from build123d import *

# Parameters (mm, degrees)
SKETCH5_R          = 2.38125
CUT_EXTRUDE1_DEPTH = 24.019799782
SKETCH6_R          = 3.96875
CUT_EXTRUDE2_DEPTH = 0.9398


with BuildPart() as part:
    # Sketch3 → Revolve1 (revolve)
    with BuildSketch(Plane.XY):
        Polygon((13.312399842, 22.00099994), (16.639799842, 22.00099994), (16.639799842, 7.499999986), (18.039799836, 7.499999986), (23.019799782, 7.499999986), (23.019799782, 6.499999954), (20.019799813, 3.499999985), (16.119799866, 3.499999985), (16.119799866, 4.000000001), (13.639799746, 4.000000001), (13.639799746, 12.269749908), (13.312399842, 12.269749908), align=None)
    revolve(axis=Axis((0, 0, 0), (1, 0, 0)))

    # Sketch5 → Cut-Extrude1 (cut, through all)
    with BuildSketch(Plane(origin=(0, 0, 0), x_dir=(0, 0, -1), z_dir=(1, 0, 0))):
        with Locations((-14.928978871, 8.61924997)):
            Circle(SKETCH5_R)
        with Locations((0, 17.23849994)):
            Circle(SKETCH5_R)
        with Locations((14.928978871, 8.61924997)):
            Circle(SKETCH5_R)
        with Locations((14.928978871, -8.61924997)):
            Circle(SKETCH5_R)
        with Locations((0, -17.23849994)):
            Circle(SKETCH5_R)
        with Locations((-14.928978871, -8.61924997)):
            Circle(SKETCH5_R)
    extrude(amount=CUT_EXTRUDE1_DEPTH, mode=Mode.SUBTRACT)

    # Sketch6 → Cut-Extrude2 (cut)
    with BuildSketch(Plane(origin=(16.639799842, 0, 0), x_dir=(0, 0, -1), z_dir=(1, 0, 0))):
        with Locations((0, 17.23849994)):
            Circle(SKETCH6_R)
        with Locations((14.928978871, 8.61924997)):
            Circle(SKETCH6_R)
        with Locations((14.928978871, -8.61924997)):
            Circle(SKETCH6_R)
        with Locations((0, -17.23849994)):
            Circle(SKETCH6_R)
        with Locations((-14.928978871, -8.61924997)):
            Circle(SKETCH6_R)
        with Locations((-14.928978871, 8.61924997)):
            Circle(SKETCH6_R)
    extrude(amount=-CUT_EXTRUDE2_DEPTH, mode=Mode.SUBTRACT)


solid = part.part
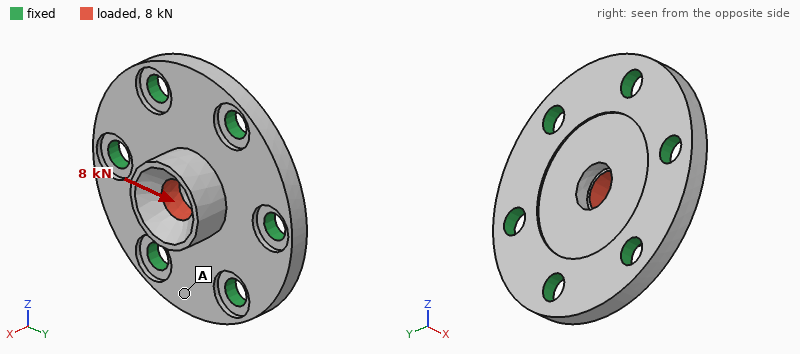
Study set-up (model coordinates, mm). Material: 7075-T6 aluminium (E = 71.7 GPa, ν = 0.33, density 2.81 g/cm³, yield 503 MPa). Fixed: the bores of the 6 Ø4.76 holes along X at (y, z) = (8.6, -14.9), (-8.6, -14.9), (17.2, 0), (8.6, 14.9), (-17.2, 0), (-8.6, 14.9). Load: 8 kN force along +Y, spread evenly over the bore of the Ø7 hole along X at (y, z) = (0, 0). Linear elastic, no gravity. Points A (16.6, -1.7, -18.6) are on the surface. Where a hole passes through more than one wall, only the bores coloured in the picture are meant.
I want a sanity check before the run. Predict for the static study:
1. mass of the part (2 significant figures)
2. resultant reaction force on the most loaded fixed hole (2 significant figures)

14 g
2.3 kN
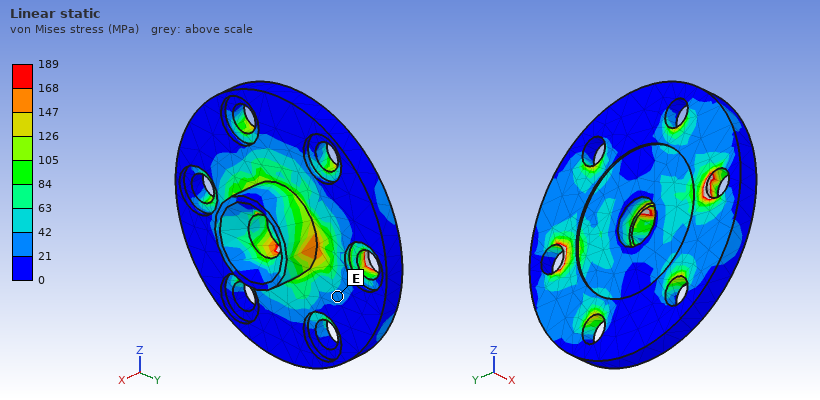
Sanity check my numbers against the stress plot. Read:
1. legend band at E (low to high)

21 to 42 MPa
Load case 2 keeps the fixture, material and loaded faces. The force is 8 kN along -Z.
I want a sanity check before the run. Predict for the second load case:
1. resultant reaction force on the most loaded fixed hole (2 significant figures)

2.0 kN
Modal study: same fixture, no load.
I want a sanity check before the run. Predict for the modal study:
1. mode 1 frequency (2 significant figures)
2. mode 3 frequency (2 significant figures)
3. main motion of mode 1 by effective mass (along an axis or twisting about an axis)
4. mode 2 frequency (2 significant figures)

23 kHz
35 kHz
along X
35 kHz
